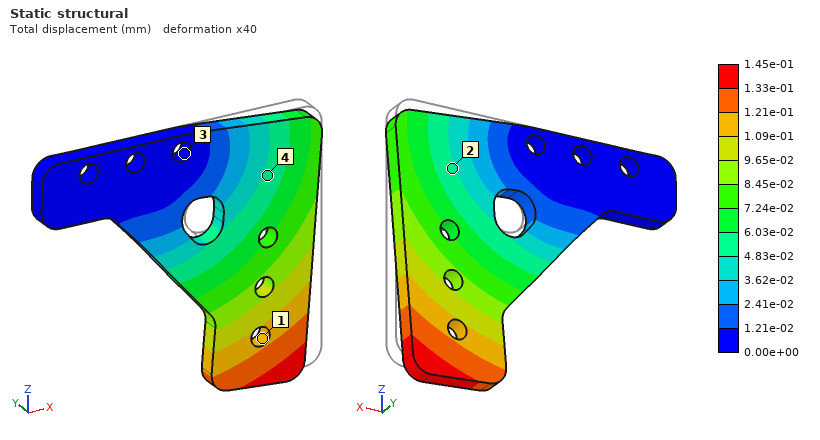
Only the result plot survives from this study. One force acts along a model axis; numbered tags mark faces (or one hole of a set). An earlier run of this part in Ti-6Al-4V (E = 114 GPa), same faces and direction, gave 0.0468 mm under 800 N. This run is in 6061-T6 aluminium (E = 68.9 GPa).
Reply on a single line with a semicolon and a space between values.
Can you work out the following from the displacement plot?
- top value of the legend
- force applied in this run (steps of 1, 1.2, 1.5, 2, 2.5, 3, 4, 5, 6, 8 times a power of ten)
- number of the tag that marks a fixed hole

1.45e-01 mm; 1.5 kN; 3
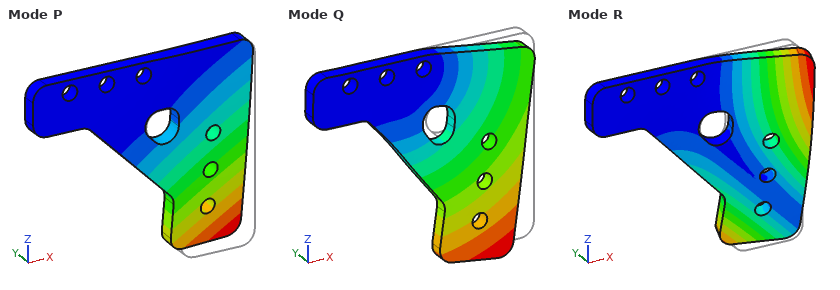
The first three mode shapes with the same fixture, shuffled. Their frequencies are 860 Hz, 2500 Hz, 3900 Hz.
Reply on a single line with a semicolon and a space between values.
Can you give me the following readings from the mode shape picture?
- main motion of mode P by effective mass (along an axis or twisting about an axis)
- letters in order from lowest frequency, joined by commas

along Y; P, R, Q
